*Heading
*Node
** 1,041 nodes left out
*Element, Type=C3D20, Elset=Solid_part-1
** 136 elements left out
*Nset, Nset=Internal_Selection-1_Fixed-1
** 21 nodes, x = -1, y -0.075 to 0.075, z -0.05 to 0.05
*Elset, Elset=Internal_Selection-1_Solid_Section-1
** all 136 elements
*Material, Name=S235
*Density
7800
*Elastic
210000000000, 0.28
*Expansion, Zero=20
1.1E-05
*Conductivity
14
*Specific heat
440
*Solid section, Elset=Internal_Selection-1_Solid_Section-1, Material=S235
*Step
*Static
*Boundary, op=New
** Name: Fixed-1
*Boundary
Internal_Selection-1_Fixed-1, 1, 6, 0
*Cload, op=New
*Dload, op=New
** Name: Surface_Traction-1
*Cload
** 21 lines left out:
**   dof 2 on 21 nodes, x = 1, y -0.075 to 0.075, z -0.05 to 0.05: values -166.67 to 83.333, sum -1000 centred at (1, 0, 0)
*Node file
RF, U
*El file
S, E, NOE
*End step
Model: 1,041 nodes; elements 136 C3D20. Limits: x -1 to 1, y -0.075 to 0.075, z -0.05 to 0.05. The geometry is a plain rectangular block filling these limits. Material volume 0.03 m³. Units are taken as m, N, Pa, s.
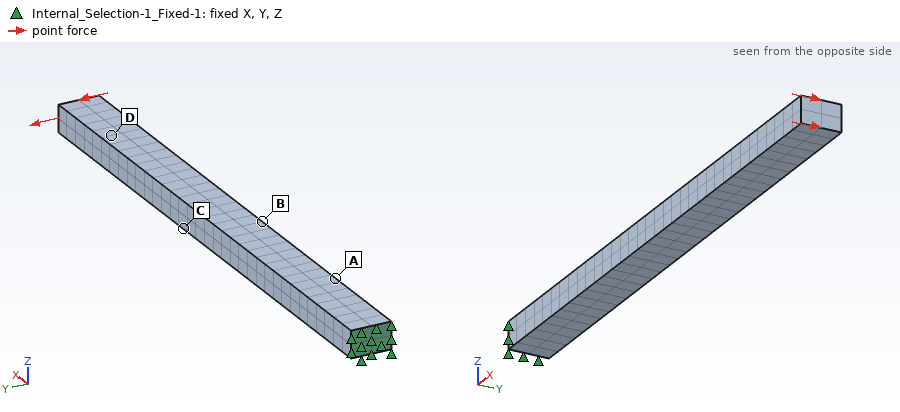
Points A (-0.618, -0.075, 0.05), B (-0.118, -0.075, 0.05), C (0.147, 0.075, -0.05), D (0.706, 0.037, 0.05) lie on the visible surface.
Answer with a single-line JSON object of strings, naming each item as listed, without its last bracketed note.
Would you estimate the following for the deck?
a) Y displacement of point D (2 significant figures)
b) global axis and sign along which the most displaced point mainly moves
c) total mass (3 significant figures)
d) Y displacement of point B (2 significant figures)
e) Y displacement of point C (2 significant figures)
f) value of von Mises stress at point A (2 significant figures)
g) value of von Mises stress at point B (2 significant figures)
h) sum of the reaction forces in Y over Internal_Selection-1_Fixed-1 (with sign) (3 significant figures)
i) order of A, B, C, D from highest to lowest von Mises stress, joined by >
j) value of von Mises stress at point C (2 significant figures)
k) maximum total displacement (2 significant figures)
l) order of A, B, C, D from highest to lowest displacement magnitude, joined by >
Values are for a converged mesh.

{"Y displacement of point D": "-3.5e-04 m", "global axis and sign along which the most displaced point mainly moves": "-Y", "total mass": "234 kg", "Y displacement of point B": "-1.1e-04 m", "Y displacement of point C": "-1.8e-04 m", "value of von Mises stress at point A": "4.3e+06 Pa", "value of von Mises stress at point B": "3.0e+06 Pa", "sum of the reaction forces in Y over Internal_Selection-1_Fixed-1 (with sign)": "1000 N", "order of A, B, C, D from highest to lowest von Mises stress, joined by >": "A > B > C > D", "value of von Mises stress at point C": "2.3e+06 Pa", "maximum total displacement": "4.5e-04 m", "order of A, B, C, D from highest to lowest displacement magnitude, joined by >": "D > C > B > A"}
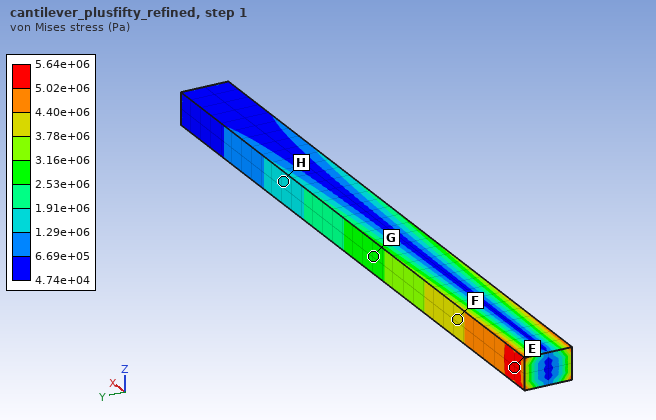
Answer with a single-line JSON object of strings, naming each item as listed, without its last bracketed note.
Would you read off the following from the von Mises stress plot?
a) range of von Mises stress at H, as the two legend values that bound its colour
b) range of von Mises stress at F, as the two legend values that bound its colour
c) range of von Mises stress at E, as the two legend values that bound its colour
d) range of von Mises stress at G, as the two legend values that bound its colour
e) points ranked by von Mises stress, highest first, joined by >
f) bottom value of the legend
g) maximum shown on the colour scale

{"range of von Mises stress at H, as the two legend values that bound its colour": "1.29e+06 to 1.91e+06 Pa", "range of von Mises stress at F, as the two legend values that bound its colour": "3.78e+06 to 4.40e+06 Pa", "range of von Mises stress at E, as the two legend values that bound its colour": "5.02e+06 to 5.64e+06 Pa", "range of von Mises stress at G, as the two legend values that bound its colour": "2.53e+06 to 3.16e+06 Pa", "points ranked by von Mises stress, highest first, joined by >": "E > F > G > H", "bottom value of the legend": "4.74e+04 Pa", "maximum shown on the colour scale": "5.64e+06 Pa"}
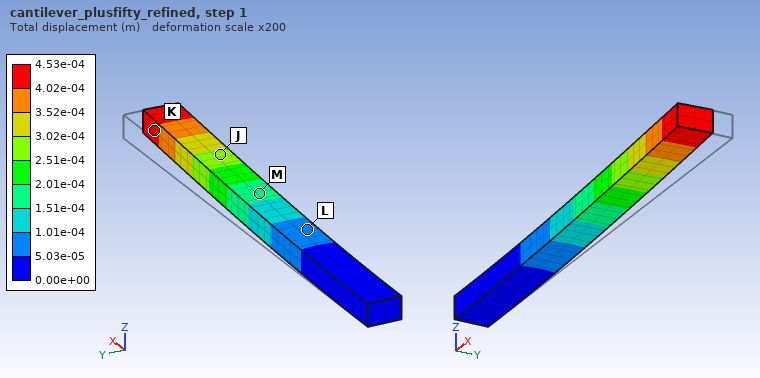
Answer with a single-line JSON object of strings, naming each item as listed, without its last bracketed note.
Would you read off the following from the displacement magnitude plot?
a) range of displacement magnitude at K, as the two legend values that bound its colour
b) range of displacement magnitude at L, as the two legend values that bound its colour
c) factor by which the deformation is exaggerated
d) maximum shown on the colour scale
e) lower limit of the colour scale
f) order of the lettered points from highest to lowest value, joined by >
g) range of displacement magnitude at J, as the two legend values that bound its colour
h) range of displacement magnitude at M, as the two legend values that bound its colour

{"range of displacement magnitude at K, as the two legend values that bound its colour": "4.02e-04 to 4.53e-04 m", "range of displacement magnitude at L, as the two legend values that bound its colour": "5.03e-05 to 1.01e-04 m", "factor by which the deformation is exaggerated": "200", "maximum shown on the colour scale": "4.53e-04 m", "lower limit of the colour scale": "0.00e+00 m", "order of the lettered points from highest to lowest value, joined by >": "K > J > M > L", "range of displacement magnitude at J, as the two legend values that bound its colour": "2.51e-04 to 3.02e-04 m", "range of displacement magnitude at M, as the two legend values that bound its colour": "1.51e-04 to 2.01e-04 m"}
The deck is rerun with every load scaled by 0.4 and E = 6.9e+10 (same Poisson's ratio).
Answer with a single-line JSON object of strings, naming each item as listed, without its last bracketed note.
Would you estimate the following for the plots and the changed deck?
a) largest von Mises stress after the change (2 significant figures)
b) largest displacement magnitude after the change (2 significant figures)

{"largest von Mises stress after the change": "2.3e+06 Pa", "largest displacement magnitude after the change": "5.5e-04 m"}
